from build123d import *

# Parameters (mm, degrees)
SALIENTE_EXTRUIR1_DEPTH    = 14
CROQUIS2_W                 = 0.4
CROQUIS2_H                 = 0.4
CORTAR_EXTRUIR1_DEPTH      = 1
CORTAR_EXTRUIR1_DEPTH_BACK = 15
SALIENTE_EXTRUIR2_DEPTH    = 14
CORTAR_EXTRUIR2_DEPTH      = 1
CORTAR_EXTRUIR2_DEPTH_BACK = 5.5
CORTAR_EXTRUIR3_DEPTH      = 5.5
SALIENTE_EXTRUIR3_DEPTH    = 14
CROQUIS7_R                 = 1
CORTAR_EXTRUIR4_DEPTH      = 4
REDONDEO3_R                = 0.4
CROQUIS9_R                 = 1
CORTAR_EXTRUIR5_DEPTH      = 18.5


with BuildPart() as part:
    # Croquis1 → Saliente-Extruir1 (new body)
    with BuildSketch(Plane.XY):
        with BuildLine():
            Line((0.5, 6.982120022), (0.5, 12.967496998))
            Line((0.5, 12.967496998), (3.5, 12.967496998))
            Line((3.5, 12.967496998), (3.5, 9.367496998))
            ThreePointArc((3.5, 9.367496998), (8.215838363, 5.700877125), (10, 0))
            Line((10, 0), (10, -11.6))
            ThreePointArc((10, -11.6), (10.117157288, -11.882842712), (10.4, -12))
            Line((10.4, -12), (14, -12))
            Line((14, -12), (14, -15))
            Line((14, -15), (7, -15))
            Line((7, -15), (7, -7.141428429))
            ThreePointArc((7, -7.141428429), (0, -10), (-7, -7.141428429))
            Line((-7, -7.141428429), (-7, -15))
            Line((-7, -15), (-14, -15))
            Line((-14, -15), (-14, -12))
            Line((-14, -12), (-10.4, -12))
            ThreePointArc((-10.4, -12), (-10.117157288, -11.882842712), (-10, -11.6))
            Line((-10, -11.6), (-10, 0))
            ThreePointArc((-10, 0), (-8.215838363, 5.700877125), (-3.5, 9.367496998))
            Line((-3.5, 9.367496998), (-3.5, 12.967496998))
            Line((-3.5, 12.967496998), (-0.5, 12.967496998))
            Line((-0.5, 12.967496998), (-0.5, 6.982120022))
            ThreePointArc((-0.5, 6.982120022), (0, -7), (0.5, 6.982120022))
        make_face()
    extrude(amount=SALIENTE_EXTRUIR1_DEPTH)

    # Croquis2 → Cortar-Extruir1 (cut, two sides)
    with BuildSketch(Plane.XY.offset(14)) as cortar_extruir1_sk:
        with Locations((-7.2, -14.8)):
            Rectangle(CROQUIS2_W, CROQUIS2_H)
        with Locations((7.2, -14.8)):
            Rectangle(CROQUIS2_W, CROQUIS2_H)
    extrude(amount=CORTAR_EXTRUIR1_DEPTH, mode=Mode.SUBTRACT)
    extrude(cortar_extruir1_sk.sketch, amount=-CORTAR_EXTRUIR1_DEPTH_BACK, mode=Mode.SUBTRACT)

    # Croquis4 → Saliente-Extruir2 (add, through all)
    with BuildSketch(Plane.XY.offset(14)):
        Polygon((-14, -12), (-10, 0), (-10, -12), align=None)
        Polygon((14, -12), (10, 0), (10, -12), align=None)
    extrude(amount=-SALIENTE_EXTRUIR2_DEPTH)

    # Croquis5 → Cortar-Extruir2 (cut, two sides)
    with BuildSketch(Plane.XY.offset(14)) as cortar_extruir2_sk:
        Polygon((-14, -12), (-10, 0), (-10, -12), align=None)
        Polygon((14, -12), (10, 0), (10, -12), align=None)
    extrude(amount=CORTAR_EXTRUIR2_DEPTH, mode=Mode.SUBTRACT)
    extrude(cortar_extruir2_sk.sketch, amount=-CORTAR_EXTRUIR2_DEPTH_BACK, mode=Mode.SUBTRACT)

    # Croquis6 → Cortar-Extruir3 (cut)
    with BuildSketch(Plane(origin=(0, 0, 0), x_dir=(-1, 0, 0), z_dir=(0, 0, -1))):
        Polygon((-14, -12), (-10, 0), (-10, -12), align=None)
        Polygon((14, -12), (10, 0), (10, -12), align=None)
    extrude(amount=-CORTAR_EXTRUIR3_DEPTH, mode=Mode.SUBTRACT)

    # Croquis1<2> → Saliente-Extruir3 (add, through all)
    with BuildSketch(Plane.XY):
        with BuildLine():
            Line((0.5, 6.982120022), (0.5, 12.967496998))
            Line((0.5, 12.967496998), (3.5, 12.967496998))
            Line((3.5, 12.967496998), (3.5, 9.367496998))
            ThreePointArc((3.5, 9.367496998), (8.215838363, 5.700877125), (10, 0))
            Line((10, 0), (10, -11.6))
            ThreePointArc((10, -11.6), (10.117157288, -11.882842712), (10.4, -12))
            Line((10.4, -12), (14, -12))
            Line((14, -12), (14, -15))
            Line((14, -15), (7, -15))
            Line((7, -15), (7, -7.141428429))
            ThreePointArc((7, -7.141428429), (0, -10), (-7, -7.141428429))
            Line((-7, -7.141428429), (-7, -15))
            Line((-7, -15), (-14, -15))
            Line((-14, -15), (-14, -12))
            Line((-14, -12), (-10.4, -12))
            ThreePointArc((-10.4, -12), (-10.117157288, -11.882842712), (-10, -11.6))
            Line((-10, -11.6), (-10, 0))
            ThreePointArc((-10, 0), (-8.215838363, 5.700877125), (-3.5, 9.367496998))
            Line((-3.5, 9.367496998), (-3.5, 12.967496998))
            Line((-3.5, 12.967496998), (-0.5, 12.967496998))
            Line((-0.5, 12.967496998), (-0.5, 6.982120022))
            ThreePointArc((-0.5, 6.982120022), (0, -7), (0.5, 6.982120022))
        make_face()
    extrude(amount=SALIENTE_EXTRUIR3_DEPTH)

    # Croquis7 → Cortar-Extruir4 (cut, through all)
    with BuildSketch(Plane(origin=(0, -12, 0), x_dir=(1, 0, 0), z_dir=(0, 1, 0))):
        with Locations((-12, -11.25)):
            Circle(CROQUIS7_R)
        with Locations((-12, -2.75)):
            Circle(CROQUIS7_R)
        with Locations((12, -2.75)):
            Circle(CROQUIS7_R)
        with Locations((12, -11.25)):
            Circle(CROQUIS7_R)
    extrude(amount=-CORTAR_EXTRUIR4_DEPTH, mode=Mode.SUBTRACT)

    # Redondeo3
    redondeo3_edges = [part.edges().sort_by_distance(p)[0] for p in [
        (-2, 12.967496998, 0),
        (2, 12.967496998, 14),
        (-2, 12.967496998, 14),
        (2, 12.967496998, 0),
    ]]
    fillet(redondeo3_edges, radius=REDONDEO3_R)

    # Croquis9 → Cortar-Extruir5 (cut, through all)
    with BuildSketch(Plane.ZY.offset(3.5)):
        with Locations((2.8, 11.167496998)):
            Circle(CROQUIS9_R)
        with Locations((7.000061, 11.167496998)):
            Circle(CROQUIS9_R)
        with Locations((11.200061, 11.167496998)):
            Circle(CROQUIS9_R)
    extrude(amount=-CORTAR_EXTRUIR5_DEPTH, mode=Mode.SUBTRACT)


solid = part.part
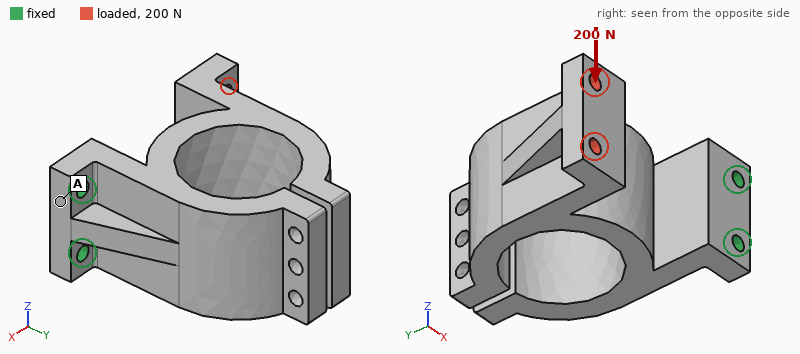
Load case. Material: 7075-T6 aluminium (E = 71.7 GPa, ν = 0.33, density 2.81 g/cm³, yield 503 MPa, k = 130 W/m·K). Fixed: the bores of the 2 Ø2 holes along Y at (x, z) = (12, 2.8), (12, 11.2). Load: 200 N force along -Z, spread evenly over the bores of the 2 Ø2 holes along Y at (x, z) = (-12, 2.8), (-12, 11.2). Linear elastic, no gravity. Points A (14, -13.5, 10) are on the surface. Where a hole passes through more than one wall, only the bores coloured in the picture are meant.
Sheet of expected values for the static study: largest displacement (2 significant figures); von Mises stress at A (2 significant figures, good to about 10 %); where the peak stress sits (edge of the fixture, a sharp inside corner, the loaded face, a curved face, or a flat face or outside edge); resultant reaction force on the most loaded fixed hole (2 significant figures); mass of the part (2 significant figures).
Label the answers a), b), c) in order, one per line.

a) 0.16 mm
b) 13 MPa
c) a curved face
d) 500 N
e) 10 g
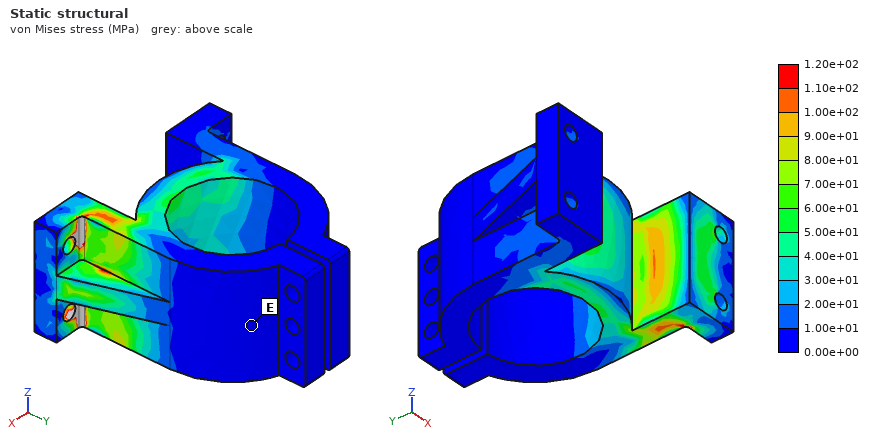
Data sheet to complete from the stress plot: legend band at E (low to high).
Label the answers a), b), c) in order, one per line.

a) 0.00e+00 to 1.00e+01 MPa
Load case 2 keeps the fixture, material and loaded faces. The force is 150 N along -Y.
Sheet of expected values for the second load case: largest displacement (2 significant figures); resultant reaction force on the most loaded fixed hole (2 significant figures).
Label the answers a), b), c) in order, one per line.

a) 0.44 mm
b) 91 N
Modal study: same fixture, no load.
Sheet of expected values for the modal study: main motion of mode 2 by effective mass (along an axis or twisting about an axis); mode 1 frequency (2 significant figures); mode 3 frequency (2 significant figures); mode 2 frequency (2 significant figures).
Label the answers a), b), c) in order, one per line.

a) along Z
b) 1600 Hz
c) 4300 Hz
d) 3200 Hz
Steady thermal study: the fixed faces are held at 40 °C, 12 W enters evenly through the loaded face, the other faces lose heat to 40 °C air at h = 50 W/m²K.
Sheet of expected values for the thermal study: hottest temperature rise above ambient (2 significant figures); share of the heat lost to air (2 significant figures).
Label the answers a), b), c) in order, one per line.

a) 58 K
b) 32 %
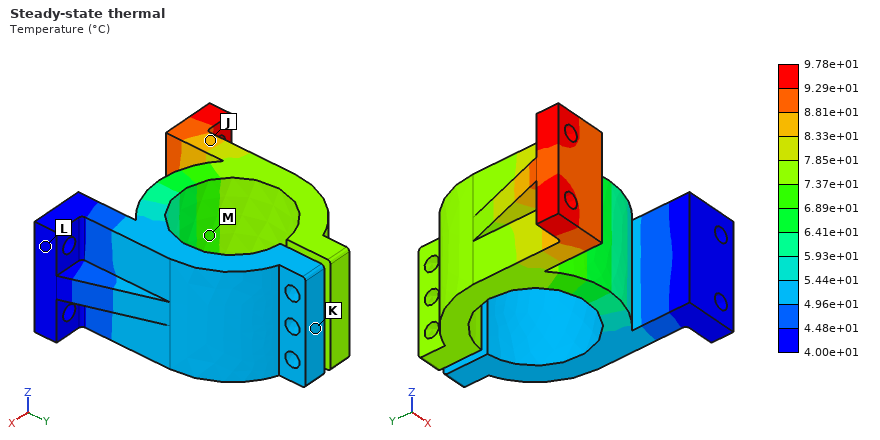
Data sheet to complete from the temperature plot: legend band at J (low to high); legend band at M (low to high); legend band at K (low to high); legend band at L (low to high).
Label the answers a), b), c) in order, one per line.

a) 8.33e+01 to 8.81e+01 °C
b) 6.89e+01 to 7.37e+01 °C
c) 4.96e+01 to 5.44e+01 °C
d) 4.00e+01 to 4.48e+01 °C
